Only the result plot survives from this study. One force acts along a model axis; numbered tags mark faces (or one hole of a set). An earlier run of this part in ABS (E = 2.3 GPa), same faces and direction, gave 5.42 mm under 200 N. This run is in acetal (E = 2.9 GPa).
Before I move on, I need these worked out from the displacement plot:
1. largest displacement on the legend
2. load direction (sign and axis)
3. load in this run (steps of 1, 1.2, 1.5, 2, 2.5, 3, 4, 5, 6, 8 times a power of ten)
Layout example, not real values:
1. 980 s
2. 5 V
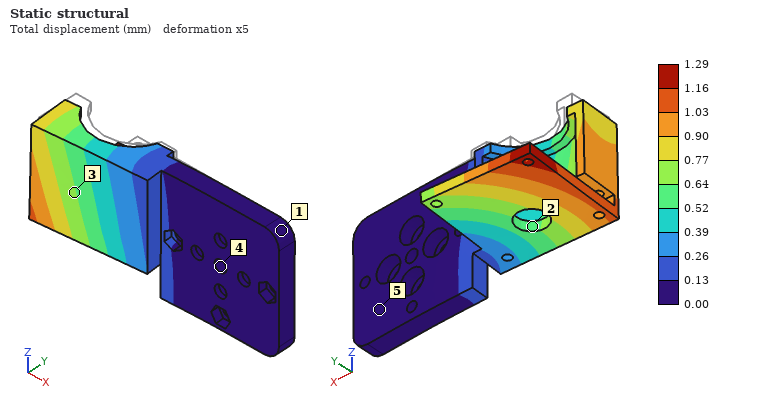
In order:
1. 1.29 mm
2. -Y
3. 60 N
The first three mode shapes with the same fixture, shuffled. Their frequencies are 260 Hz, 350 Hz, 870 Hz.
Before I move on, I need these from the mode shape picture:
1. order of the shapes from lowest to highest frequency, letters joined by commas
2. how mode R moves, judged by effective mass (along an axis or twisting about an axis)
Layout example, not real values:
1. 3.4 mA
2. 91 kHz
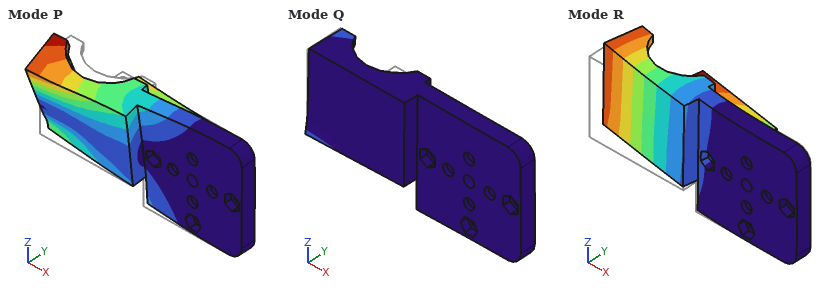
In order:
1. R, Q, P
2. along Y
